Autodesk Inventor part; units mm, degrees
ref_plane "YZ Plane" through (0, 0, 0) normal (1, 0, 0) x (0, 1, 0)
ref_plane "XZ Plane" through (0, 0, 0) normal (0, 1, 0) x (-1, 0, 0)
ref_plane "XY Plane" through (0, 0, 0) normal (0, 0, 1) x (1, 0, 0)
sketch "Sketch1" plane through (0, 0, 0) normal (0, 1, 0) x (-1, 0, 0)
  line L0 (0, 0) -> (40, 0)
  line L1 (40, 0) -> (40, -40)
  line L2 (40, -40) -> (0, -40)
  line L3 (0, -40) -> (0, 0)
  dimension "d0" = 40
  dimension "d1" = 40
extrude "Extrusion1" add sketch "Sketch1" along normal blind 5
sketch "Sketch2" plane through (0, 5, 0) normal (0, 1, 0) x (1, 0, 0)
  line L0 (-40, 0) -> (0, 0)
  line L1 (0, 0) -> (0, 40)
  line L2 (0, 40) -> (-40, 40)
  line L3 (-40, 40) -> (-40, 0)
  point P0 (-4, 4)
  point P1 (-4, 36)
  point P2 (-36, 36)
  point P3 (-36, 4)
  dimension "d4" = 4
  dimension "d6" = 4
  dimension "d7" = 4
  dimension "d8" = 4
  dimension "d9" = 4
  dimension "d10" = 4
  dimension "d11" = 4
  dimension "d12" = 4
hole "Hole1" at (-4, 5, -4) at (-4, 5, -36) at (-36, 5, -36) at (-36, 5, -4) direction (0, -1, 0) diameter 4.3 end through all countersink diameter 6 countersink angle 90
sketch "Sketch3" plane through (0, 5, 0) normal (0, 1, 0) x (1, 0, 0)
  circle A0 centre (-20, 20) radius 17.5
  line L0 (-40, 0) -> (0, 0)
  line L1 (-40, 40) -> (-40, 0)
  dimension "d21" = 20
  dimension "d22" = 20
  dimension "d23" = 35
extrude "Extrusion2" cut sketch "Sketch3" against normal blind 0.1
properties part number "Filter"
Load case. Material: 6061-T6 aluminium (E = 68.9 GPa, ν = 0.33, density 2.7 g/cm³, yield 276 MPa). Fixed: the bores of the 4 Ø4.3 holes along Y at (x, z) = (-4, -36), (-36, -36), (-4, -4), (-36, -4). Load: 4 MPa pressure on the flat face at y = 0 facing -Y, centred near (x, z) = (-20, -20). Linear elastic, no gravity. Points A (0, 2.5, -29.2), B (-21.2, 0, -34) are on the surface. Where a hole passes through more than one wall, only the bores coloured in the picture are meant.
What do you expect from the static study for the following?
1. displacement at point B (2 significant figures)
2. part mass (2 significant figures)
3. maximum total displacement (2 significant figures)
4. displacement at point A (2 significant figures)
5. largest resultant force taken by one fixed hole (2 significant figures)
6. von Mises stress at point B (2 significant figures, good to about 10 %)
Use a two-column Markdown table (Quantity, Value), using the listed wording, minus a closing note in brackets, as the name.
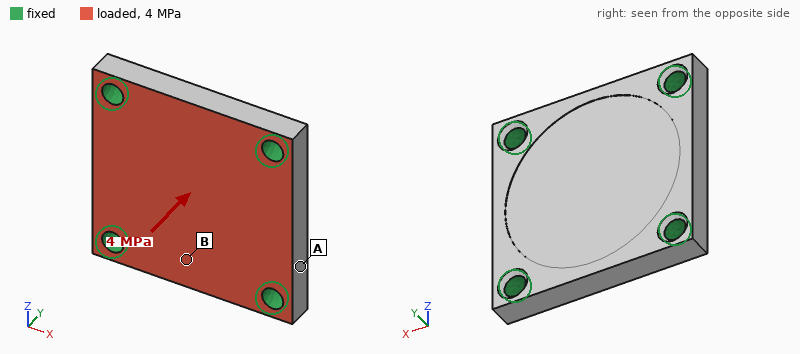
| Quantity | Value |
|---|---|
| displacement at point B | 27 µm |
| part mass | 20 g |
| maximum total displacement | 42 µm |
| displacement at point A | 6.9 µm |
| largest resultant force taken by one fixed hole | 1.5 kN |
| von Mises stress at point B | 44 MPa |
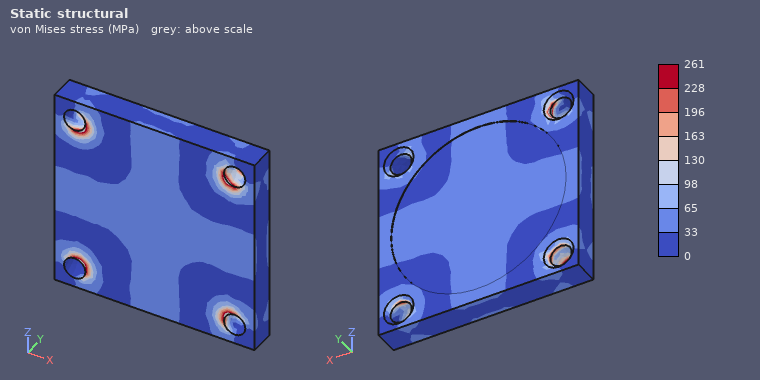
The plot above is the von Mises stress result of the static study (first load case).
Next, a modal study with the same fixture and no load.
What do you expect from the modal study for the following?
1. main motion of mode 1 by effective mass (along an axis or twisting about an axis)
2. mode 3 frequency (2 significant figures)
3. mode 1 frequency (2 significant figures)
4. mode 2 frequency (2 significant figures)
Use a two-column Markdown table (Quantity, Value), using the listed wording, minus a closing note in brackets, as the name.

| Quantity | Value |
|---|---|
| main motion of mode 1 by effective mass | along Y |
| mode 3 frequency | 26 kHz |
| mode 1 frequency | 16 kHz |
| mode 2 frequency | 26 kHz |
